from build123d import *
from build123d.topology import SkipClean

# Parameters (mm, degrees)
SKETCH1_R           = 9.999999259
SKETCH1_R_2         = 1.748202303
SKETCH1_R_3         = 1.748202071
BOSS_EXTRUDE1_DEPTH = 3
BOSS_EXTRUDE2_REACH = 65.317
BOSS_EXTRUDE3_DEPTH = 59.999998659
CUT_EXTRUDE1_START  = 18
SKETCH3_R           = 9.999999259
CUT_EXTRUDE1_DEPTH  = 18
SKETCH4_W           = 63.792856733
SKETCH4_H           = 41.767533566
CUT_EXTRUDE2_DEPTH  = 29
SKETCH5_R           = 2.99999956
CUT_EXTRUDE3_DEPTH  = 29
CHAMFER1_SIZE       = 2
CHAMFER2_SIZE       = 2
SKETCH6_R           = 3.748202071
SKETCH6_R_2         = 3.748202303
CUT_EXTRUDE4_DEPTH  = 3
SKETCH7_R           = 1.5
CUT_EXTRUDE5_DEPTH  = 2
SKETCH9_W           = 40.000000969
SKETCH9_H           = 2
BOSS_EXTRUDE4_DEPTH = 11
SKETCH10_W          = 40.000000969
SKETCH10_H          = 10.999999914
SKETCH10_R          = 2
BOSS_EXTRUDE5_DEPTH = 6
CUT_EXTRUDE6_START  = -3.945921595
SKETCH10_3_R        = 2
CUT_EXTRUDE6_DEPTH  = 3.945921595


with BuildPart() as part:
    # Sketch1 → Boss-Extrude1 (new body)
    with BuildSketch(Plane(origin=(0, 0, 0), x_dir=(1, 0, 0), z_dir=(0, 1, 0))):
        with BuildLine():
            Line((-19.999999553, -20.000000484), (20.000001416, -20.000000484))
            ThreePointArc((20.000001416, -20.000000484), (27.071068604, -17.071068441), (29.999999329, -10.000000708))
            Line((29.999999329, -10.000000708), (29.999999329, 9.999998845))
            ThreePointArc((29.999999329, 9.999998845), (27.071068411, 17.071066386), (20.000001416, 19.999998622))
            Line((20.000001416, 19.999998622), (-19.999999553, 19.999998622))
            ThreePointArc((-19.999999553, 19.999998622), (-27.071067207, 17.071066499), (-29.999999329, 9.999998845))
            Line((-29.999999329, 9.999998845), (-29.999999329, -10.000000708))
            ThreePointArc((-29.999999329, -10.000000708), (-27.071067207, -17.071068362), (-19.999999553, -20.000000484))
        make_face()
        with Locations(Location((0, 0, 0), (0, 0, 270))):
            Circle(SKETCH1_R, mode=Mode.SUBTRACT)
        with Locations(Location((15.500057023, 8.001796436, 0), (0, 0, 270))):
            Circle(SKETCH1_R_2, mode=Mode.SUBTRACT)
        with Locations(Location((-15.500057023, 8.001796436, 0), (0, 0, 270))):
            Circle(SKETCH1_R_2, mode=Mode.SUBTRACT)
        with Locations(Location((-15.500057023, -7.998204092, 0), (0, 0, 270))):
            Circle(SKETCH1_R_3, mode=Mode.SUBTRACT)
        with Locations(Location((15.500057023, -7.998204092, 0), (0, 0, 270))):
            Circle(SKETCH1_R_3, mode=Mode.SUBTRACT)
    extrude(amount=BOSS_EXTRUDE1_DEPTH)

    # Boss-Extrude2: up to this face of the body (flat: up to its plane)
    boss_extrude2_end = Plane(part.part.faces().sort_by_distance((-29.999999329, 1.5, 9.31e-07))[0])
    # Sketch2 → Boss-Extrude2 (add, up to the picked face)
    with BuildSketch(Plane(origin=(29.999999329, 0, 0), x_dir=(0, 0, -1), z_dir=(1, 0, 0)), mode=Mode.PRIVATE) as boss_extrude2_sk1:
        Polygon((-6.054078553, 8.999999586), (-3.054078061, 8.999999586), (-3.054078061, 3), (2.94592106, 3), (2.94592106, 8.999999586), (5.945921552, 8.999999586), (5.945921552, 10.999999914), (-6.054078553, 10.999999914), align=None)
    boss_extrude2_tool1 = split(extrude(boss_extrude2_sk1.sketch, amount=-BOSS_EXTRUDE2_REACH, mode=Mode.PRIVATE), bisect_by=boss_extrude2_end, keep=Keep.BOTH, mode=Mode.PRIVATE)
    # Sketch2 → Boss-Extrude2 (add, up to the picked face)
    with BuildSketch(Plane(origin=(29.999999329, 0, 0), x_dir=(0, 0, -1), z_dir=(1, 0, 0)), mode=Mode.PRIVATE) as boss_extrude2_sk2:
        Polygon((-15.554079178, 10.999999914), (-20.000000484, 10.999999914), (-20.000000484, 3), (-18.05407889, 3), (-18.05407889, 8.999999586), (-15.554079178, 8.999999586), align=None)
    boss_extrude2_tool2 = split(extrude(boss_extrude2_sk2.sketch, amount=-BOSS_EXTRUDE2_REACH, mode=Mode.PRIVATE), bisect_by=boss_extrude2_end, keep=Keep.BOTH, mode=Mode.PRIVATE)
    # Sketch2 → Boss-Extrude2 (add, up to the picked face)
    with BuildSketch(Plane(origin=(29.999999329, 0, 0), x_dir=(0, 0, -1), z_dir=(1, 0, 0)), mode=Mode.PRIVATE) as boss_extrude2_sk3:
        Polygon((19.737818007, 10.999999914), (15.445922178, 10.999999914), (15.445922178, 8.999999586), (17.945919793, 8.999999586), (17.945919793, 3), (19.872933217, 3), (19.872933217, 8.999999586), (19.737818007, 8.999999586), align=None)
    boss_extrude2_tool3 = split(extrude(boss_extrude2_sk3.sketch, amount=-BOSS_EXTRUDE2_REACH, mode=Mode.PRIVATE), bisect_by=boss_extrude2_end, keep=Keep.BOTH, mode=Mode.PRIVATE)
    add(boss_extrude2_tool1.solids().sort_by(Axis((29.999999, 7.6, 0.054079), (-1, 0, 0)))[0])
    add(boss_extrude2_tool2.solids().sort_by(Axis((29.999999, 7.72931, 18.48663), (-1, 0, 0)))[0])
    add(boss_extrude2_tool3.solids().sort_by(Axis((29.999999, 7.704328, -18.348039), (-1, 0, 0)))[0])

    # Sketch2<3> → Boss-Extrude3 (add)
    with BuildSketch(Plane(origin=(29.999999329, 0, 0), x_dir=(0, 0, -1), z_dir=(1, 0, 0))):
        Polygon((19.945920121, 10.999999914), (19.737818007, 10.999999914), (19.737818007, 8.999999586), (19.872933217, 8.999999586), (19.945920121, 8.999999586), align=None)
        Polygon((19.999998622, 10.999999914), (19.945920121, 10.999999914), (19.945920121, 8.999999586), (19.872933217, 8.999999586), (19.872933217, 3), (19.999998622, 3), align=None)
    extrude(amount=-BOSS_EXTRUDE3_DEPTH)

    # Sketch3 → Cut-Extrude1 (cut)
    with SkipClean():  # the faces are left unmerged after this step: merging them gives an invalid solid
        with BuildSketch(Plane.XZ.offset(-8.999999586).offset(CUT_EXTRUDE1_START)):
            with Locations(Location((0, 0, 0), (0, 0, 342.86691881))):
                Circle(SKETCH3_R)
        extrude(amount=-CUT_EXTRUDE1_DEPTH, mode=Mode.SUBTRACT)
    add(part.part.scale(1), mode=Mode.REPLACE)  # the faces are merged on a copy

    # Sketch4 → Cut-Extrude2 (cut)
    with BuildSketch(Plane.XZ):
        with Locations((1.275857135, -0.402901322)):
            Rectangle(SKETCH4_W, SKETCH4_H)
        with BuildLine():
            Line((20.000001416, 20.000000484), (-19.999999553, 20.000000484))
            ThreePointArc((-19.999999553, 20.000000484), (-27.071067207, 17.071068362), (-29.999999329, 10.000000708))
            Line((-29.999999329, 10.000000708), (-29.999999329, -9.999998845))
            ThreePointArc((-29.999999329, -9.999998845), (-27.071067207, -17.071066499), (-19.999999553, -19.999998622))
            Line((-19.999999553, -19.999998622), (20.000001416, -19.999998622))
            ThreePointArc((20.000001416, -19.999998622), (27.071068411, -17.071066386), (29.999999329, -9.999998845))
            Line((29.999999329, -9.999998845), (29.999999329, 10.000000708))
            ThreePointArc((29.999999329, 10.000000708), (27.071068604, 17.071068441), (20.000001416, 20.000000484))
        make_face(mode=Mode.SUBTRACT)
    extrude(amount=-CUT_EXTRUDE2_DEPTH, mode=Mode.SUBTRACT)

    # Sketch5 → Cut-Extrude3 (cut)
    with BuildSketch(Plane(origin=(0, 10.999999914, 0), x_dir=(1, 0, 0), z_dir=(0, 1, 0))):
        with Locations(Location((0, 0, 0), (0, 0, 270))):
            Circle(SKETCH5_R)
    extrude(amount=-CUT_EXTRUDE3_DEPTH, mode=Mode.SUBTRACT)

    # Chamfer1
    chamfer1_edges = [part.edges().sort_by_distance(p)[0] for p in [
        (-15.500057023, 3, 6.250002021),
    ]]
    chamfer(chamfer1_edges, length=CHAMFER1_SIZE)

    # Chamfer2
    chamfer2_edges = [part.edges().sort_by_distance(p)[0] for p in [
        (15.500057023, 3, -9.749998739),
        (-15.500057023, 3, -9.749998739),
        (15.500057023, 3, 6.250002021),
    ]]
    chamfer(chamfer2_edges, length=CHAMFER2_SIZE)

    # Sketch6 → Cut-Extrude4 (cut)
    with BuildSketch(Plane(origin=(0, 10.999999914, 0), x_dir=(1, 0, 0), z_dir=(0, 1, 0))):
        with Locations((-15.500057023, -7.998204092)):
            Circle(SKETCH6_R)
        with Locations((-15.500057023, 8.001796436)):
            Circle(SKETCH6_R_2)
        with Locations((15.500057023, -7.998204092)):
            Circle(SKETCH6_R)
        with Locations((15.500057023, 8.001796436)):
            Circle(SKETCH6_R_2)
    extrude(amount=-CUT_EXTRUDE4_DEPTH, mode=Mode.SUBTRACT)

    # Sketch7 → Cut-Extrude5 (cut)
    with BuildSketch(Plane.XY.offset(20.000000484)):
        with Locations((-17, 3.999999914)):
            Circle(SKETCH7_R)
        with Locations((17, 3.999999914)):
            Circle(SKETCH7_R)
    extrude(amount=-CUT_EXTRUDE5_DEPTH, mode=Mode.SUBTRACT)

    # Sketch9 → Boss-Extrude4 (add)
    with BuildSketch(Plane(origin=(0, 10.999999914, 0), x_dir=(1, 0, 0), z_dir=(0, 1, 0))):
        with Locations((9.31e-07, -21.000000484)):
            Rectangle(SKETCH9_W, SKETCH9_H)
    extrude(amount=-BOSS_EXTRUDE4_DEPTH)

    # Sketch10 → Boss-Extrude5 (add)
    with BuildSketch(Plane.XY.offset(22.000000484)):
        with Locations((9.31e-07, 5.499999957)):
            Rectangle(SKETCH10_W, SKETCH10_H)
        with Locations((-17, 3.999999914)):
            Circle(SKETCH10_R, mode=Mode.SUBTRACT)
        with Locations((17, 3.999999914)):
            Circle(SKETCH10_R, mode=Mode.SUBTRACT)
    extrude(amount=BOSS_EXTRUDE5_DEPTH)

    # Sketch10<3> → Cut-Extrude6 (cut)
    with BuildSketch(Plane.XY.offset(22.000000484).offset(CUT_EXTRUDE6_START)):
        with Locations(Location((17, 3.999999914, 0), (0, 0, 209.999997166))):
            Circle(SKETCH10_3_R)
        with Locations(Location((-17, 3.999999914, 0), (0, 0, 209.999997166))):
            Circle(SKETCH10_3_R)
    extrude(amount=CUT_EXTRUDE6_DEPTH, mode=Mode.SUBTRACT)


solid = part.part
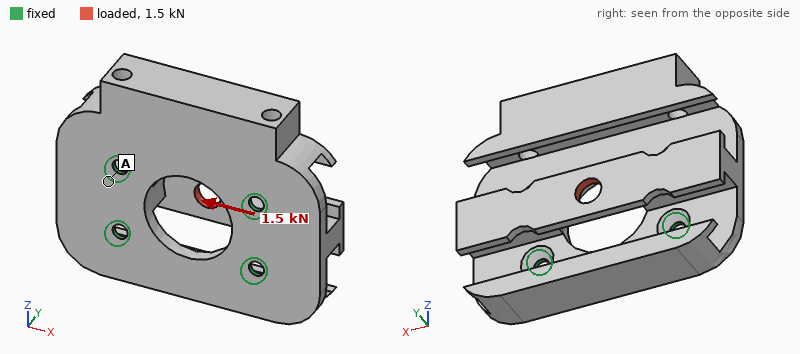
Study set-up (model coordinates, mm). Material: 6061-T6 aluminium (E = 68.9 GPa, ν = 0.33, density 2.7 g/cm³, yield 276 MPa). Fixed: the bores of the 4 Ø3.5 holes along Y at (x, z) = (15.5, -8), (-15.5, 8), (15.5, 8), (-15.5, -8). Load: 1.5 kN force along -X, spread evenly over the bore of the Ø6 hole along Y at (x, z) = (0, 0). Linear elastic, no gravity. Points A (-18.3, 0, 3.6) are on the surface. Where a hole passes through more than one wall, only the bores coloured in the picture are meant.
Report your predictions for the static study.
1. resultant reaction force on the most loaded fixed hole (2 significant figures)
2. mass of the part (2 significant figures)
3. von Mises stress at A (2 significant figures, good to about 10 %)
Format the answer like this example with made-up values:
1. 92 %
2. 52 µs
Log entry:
1. 450 N
2. 38 g
3. 24 MPa
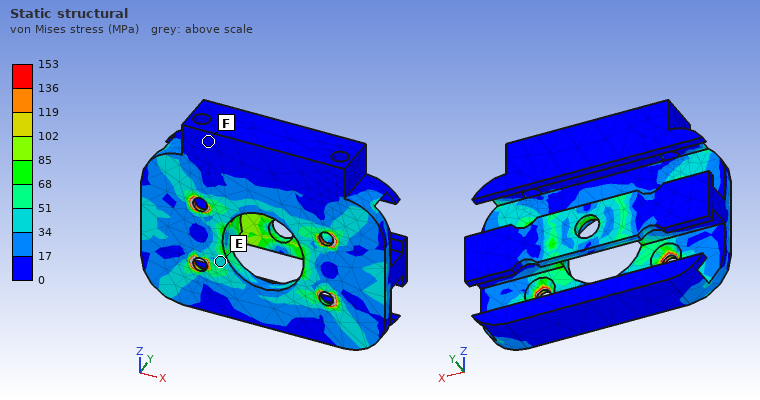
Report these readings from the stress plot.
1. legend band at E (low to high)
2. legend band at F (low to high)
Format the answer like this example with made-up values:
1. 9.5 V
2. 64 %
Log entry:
1. 34 to 51 MPa
2. 0 to 17 MPa
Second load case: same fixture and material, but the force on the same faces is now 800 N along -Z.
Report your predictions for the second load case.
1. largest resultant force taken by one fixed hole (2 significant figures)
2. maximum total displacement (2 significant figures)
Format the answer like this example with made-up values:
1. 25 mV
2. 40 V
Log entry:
1. 340 N
2. 36 µm
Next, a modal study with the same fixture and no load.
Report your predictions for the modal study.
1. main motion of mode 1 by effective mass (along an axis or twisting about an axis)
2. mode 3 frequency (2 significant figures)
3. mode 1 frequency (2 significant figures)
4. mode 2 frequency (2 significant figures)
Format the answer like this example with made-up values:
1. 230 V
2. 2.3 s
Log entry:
1. along Y
2. 6700 Hz
3. 2500 Hz
4. 5700 Hz
